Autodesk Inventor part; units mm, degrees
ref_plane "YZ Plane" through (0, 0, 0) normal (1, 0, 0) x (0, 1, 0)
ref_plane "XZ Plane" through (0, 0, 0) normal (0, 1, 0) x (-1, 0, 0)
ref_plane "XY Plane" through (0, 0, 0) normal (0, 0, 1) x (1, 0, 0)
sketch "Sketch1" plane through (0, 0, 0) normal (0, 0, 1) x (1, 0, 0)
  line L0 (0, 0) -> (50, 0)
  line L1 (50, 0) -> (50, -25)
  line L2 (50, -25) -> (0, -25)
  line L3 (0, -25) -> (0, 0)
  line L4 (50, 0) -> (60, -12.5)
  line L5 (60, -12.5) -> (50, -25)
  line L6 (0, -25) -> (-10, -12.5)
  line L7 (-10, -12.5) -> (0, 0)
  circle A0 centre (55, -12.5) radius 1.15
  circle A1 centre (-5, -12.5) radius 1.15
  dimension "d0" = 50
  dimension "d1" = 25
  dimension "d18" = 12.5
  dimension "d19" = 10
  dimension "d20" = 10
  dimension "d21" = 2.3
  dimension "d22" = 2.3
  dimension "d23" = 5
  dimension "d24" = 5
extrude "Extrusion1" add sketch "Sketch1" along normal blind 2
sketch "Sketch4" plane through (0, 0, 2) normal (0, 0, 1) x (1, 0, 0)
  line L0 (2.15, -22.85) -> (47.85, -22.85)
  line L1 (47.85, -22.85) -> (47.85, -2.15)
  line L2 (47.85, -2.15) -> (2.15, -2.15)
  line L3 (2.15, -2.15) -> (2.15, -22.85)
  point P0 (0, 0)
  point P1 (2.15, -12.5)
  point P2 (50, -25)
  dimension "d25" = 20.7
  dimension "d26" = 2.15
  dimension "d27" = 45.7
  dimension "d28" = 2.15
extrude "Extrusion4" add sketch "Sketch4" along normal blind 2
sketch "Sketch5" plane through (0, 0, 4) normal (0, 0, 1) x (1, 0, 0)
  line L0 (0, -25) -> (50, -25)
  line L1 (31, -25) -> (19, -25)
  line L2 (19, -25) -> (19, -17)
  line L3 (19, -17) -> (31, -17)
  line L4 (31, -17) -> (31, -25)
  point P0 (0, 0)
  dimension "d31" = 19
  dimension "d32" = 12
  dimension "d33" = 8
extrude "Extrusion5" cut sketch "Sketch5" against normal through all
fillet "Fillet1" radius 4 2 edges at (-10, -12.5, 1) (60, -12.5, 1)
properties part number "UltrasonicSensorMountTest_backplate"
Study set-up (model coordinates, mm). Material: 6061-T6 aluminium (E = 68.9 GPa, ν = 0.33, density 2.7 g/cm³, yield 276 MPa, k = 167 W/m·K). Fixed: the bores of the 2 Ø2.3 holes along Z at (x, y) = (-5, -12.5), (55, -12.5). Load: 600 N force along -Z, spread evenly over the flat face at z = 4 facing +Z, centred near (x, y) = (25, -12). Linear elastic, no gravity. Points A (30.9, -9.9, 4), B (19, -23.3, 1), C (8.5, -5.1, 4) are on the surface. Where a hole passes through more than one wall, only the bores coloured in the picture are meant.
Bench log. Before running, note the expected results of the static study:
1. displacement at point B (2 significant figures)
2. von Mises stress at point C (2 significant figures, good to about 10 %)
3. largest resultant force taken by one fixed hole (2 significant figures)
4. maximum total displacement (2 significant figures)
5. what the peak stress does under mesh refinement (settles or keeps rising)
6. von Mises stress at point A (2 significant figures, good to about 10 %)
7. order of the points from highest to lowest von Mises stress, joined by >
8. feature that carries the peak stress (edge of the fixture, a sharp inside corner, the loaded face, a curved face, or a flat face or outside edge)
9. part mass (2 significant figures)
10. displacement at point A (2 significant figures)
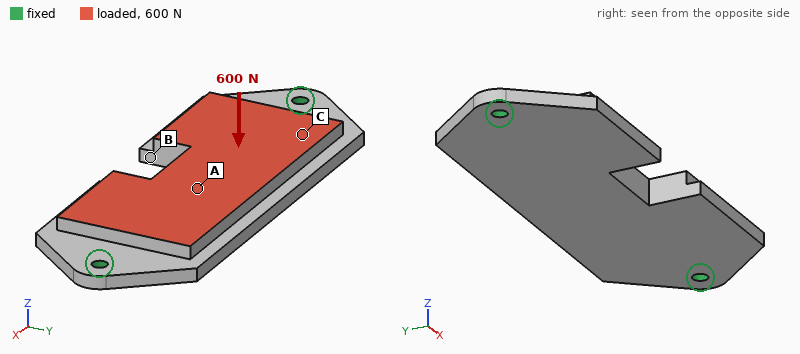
0.15 mm
37 MPa
680 N
0.18 mm
keeps rising
75 MPa
A > C > B
edge of the fixture
12 g
0.15 mm
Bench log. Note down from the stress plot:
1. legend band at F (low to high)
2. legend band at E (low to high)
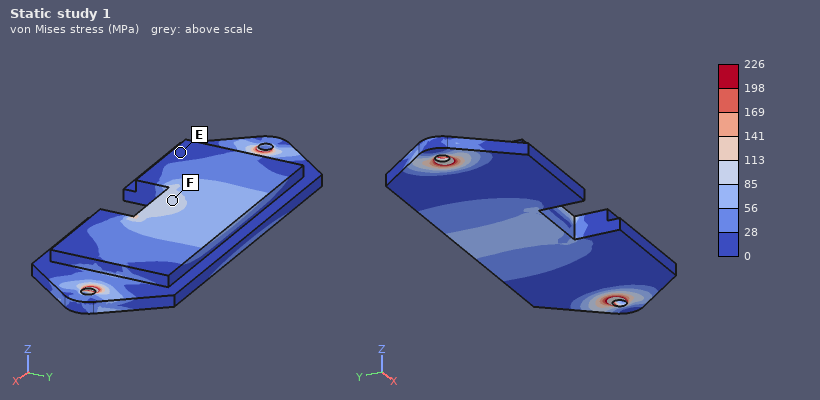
85 to 113 MPa
0 to 28 MPa
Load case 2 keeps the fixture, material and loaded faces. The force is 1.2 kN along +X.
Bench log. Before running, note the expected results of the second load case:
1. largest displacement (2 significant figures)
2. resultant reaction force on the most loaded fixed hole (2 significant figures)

7.1 µm
600 N
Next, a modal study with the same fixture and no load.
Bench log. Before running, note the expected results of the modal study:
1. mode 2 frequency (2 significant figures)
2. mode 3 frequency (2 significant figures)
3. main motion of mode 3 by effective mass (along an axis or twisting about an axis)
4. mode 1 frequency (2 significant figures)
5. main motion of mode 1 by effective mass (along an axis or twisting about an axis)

3900 Hz
8600 Hz
twisting about Y
3300 Hz
along Z
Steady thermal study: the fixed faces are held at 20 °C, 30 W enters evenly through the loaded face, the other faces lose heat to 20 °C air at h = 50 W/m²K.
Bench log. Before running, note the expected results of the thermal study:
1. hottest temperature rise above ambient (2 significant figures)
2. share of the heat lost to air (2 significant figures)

35 K
11 %
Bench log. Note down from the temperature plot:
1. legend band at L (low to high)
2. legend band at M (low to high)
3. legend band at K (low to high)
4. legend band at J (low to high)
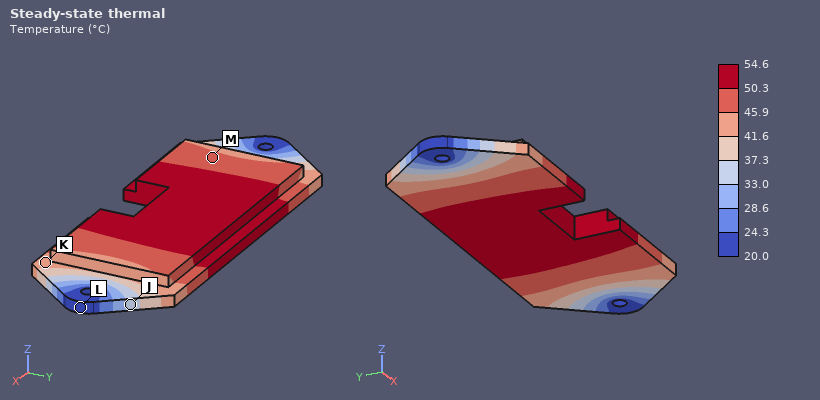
20.0 to 24.3 °C
45.9 to 50.3 °C
41.6 to 45.9 °C
33.0 to 37.3 °C
